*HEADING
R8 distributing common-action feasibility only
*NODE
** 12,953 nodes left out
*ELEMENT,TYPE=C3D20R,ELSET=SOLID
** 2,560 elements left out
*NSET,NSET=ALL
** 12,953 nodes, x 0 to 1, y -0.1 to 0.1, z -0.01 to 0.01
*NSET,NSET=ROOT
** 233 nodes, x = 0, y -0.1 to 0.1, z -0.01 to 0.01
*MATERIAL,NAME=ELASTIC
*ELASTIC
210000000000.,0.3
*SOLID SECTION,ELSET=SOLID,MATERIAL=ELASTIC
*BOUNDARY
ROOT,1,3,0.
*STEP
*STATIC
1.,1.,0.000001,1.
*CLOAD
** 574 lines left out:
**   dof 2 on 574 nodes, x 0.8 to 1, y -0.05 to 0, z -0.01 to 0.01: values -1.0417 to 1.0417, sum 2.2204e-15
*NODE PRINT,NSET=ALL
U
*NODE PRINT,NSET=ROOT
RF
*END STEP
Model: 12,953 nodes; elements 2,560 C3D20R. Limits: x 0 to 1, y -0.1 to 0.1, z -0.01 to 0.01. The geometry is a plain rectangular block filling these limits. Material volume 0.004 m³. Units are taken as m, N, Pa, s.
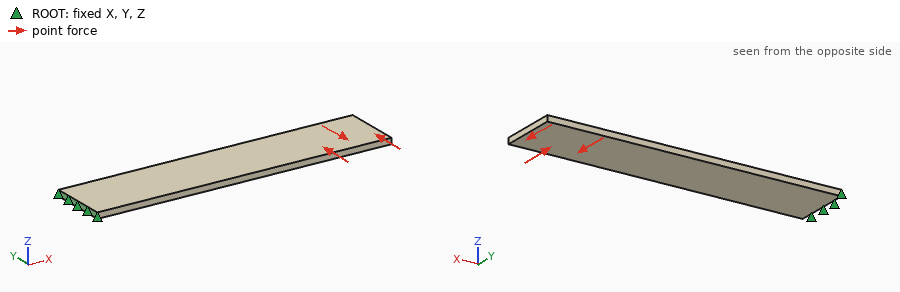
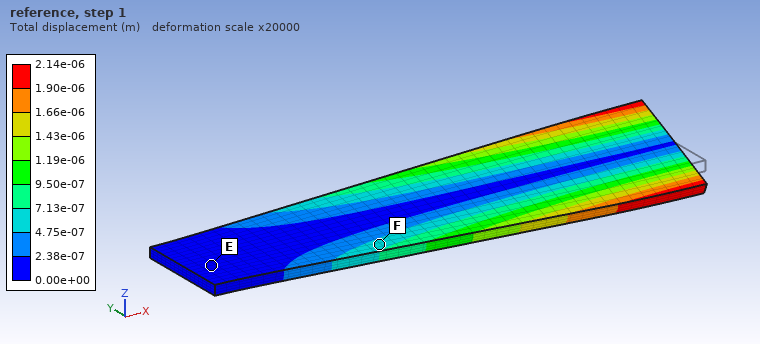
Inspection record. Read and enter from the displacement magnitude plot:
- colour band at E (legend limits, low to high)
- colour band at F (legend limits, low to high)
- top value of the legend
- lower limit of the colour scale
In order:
0.00e+00 to 2.38e-07 m
4.75e-07 to 7.13e-07 m
2.14e-06 m
0.00e+00 m
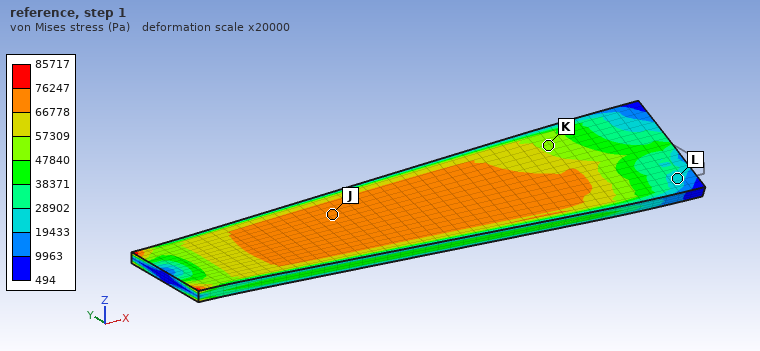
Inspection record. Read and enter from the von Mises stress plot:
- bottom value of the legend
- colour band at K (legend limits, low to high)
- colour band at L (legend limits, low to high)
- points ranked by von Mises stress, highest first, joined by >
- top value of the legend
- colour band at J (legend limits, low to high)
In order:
494 Pa
47840 to 57309 Pa
19433 to 28902 Pa
J > K > L
85717 Pa
66778 to 76247 Pa
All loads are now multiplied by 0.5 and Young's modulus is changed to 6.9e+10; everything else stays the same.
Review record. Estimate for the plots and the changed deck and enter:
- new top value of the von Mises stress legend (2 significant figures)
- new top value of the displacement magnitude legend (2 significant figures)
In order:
43000 Pa
3.3e-06 m
